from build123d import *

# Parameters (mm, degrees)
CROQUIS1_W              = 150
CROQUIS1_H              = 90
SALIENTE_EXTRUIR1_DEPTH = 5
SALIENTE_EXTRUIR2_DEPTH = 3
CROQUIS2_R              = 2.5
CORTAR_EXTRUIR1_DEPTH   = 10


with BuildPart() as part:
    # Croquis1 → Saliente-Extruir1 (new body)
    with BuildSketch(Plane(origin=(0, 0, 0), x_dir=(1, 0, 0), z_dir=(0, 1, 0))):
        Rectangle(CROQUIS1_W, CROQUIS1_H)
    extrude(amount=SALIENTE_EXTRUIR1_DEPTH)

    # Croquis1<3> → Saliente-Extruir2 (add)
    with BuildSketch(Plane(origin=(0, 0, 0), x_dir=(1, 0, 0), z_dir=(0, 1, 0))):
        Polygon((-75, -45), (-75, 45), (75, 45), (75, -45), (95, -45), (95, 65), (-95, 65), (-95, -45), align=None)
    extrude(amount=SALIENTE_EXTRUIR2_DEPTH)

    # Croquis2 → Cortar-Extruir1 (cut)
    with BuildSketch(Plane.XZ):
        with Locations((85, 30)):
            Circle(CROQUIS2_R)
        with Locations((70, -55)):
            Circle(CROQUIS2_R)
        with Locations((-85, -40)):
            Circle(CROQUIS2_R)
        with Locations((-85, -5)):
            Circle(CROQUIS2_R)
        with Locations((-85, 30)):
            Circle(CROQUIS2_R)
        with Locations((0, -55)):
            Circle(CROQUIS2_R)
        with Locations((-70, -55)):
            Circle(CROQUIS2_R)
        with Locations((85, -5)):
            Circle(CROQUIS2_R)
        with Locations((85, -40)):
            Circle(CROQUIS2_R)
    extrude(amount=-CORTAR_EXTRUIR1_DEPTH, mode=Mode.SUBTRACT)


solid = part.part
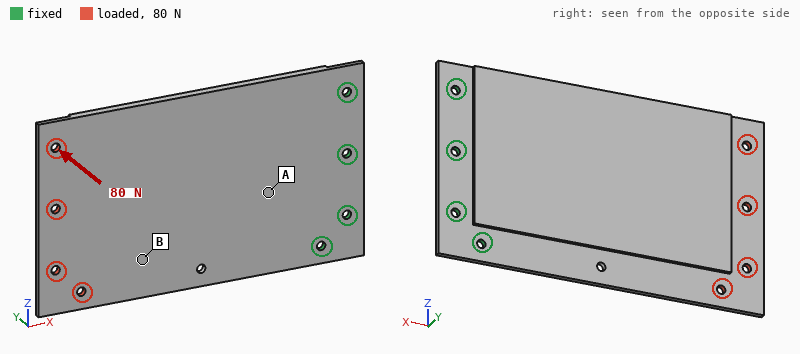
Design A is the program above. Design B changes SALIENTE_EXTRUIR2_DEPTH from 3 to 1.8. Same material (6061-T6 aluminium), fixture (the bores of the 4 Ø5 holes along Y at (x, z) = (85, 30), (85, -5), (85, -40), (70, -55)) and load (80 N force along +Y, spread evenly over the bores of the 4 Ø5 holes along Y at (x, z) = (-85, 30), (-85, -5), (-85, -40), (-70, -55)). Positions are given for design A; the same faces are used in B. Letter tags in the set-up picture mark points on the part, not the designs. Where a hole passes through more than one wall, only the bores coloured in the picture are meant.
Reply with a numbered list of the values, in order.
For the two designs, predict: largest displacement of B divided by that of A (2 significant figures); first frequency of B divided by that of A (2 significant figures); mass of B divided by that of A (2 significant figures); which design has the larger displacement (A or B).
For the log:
1. 2.0
2. 0.73
3. 0.90
4. B
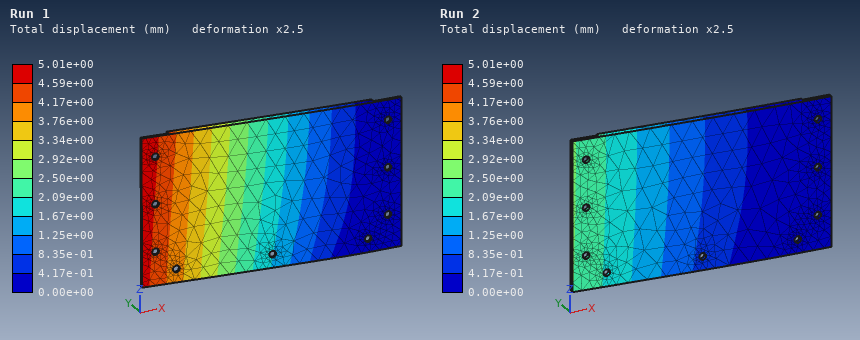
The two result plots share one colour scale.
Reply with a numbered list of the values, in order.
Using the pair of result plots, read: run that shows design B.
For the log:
1. Run 1
